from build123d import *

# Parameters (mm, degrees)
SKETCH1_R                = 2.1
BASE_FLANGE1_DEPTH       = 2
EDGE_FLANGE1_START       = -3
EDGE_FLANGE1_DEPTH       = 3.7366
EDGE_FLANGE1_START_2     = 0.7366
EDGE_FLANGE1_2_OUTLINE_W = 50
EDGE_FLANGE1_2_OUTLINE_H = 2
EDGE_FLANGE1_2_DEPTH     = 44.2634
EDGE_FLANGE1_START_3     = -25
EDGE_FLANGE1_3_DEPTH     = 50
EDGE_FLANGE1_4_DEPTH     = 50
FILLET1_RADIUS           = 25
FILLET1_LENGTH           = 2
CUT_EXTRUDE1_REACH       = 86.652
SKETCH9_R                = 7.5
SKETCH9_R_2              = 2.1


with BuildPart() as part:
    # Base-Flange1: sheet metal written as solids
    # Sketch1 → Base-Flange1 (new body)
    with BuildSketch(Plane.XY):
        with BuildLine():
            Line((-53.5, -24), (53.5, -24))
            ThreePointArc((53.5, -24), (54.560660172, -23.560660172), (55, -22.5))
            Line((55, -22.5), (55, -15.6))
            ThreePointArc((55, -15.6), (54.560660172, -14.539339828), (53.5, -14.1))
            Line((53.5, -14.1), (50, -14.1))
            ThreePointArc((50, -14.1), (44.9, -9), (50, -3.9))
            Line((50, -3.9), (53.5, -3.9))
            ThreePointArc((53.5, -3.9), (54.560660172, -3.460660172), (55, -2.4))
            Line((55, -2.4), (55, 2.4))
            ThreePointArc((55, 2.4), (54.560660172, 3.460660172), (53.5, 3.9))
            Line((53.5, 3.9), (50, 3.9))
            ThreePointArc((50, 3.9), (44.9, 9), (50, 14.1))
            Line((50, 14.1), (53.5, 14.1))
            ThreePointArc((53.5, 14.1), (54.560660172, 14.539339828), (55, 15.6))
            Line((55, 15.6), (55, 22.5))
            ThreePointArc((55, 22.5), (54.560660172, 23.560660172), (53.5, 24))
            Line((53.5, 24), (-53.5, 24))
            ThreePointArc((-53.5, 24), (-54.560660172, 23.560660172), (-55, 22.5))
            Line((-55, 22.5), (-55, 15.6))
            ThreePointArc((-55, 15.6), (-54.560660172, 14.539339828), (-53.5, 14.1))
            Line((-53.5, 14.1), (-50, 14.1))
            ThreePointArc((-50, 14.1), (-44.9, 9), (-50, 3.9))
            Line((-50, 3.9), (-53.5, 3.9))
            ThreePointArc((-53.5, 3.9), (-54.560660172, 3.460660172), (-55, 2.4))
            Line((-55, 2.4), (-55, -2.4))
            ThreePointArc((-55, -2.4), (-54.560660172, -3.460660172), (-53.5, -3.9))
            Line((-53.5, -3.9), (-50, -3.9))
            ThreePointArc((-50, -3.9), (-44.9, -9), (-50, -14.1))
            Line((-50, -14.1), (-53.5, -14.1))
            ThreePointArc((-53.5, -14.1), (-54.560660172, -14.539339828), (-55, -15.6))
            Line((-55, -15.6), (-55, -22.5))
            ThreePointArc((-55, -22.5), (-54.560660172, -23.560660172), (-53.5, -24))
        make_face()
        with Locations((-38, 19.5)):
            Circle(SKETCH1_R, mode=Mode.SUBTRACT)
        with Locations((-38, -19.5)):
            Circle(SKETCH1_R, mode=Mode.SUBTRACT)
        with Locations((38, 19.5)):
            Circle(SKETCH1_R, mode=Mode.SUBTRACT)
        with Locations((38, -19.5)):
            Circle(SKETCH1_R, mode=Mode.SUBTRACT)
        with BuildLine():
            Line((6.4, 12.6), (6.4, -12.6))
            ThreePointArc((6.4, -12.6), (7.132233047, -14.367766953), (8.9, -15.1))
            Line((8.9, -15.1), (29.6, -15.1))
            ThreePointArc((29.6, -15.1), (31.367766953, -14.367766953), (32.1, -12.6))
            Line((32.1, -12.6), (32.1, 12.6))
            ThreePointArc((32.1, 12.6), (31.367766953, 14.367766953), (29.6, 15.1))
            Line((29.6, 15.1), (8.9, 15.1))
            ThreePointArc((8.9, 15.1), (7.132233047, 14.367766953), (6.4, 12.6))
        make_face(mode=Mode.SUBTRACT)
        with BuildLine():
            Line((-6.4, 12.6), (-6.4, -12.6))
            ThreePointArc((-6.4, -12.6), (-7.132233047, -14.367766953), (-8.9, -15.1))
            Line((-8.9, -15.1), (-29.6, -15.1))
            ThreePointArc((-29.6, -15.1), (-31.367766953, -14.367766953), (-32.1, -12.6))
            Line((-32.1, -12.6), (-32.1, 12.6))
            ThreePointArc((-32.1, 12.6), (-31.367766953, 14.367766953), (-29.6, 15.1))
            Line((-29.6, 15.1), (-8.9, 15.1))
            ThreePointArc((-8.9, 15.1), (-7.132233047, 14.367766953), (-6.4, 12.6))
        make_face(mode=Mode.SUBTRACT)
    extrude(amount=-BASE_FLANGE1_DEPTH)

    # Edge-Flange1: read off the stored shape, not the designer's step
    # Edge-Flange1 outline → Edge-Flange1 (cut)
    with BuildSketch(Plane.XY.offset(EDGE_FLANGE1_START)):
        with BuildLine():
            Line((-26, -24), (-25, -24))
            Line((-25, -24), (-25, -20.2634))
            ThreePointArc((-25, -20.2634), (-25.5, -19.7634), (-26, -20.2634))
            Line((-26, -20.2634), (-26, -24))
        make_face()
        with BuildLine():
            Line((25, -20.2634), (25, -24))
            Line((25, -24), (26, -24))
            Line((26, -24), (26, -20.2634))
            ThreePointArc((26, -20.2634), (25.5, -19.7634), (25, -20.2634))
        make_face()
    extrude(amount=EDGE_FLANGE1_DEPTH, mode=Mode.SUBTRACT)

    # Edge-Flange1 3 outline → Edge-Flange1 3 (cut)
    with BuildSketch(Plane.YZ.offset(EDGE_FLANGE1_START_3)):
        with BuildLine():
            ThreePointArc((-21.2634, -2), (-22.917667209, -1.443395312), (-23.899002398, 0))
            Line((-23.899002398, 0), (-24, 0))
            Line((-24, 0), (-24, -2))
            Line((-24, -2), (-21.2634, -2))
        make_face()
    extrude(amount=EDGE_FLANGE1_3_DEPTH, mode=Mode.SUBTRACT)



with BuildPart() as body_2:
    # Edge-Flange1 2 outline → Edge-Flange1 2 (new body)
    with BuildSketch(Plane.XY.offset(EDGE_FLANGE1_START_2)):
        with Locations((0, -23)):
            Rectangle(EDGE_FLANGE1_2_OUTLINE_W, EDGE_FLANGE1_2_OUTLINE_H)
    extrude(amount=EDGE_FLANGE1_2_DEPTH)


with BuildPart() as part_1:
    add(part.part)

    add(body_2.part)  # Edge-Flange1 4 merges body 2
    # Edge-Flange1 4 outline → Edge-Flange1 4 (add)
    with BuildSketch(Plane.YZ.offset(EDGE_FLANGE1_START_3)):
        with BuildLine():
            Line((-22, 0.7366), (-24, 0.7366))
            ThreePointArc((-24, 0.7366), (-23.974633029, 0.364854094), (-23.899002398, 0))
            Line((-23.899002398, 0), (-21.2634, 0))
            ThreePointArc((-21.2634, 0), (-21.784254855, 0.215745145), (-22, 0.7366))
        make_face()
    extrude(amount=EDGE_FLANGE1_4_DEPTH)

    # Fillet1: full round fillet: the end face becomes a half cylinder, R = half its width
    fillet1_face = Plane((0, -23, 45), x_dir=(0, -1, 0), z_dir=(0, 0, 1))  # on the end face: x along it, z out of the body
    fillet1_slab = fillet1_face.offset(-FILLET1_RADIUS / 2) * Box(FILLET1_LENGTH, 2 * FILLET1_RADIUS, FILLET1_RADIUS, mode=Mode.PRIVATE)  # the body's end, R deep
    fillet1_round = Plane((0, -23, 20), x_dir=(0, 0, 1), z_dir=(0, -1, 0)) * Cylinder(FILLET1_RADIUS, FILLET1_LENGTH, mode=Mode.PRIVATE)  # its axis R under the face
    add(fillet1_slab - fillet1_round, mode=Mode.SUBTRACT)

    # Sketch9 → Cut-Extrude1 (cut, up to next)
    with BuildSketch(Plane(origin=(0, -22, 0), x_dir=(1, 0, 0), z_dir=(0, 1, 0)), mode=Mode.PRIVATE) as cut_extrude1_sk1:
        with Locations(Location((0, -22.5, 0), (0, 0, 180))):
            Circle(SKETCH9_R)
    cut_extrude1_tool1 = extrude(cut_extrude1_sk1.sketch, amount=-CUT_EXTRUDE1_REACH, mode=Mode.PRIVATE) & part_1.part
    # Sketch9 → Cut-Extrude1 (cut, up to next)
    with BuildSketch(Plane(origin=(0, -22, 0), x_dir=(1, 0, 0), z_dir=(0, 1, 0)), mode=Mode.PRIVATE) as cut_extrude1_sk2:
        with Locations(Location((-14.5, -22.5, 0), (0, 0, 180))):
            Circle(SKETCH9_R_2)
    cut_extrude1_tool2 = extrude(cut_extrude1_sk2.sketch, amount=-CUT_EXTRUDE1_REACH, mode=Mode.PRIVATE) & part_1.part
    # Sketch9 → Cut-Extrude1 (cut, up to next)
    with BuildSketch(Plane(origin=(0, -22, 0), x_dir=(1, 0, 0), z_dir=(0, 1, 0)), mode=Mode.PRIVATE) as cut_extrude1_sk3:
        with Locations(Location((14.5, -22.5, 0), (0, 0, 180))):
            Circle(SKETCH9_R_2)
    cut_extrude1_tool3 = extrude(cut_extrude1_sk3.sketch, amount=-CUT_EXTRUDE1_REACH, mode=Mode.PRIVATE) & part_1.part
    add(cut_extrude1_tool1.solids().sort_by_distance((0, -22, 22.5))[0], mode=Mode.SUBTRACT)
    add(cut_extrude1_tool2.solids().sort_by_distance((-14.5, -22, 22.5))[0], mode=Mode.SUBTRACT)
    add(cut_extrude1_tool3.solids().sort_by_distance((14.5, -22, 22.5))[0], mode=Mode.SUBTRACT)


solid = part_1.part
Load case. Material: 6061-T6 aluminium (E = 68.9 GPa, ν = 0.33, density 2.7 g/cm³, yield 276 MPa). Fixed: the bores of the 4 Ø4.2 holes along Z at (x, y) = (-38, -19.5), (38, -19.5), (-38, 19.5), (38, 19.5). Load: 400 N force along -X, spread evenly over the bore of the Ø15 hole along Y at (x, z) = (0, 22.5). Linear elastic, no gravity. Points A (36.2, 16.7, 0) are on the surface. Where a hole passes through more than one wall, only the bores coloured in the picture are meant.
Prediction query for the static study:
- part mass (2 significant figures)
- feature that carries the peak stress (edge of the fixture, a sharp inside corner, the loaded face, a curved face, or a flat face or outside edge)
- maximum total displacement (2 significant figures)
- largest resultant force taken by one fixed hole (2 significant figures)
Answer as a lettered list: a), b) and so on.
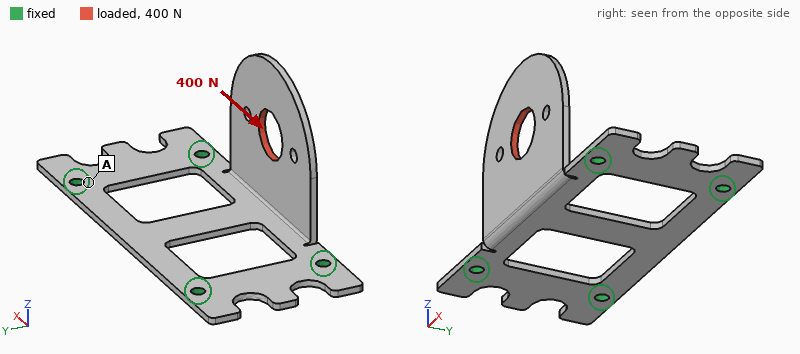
a) 27 g
b) a curved face
c) 0.33 mm
d) 250 N
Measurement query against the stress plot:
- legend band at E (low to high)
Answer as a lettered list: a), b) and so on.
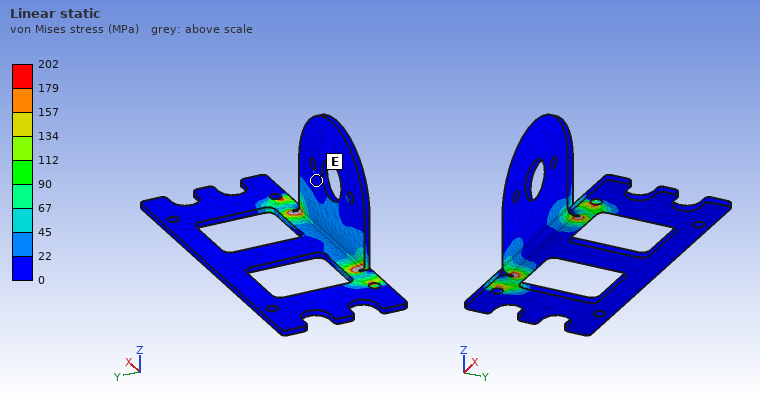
a) 0 to 22 MPa
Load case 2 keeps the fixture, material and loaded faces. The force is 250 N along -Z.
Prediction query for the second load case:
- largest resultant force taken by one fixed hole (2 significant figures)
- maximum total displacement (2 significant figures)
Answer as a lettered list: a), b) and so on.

a) 130 N
b) 0.58 mm
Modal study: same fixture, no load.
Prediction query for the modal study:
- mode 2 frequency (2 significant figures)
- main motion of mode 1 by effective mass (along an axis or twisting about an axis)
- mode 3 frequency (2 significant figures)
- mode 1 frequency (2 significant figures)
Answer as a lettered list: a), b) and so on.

a) 1800 Hz
b) along Y
c) 1800 Hz
d) 520 Hz
